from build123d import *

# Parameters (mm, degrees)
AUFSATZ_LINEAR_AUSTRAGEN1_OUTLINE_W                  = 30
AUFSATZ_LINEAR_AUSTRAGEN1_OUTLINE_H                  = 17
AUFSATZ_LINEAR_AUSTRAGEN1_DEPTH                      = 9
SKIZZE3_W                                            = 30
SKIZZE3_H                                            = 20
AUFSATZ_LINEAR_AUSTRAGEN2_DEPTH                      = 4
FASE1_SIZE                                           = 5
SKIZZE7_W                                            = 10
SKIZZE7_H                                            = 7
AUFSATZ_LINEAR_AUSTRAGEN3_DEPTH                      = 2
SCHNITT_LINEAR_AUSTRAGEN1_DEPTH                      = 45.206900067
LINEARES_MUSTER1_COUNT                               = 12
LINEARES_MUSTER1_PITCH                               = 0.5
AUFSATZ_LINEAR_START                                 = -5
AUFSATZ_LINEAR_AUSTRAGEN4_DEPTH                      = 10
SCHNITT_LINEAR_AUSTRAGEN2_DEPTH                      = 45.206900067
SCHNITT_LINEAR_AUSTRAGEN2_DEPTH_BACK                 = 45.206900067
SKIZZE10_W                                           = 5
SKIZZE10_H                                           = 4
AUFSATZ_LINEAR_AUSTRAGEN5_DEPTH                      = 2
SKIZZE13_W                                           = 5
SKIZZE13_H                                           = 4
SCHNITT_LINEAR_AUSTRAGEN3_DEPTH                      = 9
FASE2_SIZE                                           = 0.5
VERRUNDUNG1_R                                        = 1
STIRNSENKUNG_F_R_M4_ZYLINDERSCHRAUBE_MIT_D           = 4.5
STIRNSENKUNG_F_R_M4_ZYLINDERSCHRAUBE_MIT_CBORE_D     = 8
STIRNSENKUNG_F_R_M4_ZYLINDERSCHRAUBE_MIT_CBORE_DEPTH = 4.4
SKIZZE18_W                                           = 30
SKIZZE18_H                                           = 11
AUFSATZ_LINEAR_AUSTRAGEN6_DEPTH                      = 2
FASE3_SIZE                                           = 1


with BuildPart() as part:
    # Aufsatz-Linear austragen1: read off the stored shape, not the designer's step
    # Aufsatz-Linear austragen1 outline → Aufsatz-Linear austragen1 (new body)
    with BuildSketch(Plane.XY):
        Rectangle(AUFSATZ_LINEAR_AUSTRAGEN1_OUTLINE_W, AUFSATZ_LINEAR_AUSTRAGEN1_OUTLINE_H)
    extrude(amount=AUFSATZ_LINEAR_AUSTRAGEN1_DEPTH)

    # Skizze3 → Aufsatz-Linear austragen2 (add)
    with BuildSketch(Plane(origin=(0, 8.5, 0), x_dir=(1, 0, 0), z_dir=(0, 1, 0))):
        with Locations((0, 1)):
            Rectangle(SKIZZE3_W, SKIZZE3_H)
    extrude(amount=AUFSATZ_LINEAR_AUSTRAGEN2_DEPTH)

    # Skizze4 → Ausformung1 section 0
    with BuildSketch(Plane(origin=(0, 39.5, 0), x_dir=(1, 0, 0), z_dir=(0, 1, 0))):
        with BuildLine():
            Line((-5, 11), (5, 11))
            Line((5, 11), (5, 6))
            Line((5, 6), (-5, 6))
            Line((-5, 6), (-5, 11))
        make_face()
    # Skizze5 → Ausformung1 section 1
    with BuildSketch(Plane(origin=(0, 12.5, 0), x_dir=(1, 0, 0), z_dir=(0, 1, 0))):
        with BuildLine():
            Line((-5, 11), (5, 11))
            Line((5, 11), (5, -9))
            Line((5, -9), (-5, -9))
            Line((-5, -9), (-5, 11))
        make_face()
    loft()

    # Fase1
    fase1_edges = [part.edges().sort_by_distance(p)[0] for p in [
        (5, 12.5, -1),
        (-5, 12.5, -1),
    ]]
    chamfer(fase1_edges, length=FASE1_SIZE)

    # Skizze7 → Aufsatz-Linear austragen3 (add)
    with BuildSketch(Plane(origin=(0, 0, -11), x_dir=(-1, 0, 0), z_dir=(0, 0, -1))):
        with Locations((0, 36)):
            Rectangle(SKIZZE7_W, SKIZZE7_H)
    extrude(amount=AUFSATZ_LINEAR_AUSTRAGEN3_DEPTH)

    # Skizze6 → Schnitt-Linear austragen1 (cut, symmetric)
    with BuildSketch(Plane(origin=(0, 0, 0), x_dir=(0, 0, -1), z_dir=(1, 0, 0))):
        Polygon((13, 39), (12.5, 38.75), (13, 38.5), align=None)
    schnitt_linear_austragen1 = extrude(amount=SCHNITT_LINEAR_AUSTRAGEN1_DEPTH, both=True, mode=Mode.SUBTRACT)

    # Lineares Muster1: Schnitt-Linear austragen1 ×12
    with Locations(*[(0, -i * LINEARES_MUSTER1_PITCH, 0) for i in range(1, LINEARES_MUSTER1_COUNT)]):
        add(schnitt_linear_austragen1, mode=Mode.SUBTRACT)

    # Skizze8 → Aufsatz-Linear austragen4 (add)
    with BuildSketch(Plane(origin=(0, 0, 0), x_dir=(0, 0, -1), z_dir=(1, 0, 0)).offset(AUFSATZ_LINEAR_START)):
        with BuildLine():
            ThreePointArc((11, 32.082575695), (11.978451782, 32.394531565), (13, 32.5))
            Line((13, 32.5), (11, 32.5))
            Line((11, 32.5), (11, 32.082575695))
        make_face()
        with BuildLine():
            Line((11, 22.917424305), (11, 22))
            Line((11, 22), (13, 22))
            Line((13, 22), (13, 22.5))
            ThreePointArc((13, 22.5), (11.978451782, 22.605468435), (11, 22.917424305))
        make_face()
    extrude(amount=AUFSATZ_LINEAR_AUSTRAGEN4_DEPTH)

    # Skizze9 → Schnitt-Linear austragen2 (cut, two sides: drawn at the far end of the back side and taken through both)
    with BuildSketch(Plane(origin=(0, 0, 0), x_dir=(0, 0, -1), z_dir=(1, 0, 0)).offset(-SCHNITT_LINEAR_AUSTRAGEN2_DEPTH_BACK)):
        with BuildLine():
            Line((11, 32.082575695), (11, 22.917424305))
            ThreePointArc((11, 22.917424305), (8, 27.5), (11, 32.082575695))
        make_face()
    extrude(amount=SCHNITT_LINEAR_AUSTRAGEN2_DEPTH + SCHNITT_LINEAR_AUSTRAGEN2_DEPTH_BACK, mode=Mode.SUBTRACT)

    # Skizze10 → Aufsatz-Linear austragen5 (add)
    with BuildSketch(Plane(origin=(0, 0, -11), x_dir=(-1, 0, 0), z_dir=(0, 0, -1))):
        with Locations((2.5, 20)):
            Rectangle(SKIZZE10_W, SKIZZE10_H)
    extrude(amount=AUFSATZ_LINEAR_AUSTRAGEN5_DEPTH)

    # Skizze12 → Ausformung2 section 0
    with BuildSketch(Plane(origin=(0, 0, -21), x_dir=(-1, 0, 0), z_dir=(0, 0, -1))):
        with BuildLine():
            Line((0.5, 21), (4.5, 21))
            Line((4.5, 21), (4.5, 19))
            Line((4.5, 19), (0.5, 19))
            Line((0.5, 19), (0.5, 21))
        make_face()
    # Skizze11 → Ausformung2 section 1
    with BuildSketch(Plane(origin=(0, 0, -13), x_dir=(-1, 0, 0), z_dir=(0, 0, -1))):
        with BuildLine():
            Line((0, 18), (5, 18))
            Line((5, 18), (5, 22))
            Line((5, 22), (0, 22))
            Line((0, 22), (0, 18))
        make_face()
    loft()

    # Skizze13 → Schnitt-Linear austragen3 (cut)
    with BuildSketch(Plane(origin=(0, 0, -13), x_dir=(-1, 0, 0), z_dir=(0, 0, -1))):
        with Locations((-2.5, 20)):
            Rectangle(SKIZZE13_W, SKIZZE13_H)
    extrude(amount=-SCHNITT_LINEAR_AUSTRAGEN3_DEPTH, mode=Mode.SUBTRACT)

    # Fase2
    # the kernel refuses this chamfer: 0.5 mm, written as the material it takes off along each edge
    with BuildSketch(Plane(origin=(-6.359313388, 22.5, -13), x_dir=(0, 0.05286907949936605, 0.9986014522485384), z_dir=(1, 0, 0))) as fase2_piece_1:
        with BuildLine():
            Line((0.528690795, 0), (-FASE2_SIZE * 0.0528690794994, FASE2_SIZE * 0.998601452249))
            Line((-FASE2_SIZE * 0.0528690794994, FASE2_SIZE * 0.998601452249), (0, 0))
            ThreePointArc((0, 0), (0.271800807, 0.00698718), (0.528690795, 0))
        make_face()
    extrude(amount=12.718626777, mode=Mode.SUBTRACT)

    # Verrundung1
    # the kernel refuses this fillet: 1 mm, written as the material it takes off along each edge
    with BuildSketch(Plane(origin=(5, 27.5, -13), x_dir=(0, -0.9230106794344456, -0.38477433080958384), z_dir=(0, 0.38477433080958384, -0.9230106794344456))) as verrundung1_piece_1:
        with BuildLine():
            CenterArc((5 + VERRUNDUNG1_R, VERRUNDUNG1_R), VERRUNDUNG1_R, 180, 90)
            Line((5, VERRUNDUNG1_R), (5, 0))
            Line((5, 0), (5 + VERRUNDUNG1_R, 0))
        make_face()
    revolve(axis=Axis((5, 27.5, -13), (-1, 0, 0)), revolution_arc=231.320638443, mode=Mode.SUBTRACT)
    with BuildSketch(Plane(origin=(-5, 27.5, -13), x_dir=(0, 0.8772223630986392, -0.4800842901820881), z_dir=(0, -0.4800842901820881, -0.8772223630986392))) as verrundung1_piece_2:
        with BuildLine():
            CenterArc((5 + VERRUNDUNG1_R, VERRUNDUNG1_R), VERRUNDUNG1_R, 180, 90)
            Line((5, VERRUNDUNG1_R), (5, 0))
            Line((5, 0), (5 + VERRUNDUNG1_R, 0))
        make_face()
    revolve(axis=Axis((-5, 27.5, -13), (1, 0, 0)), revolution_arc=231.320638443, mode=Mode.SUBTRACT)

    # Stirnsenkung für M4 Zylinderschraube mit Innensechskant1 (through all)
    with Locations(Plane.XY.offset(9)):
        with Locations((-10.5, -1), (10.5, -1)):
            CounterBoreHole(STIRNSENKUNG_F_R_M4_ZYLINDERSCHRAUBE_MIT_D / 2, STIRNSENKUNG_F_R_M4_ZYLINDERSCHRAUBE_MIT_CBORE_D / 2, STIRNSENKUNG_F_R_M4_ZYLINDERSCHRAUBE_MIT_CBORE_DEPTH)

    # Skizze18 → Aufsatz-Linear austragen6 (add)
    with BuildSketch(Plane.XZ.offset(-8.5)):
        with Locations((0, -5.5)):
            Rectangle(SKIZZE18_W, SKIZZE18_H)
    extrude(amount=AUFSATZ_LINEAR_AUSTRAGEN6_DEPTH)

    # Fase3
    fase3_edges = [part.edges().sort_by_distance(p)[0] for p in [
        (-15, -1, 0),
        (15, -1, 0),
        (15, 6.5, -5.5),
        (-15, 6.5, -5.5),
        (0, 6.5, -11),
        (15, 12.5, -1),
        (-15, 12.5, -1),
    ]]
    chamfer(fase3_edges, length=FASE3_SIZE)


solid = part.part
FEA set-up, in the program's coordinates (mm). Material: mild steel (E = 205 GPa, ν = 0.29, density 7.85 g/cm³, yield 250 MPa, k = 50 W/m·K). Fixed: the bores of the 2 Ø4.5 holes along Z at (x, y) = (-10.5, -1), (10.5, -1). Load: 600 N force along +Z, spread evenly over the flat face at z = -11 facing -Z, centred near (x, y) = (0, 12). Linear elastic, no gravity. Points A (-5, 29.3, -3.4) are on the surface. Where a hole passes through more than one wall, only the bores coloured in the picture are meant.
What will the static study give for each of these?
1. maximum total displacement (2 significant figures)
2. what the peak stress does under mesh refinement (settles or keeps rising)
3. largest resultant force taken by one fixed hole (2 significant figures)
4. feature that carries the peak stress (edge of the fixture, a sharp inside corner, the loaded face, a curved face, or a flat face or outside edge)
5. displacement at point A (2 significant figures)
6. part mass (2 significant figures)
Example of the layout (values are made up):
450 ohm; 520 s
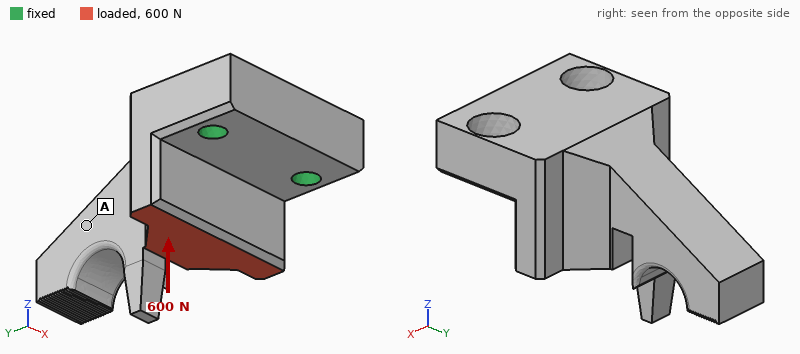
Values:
16 µm; keeps rising; 300 N; edge of the fixture; 11 µm; 85 g
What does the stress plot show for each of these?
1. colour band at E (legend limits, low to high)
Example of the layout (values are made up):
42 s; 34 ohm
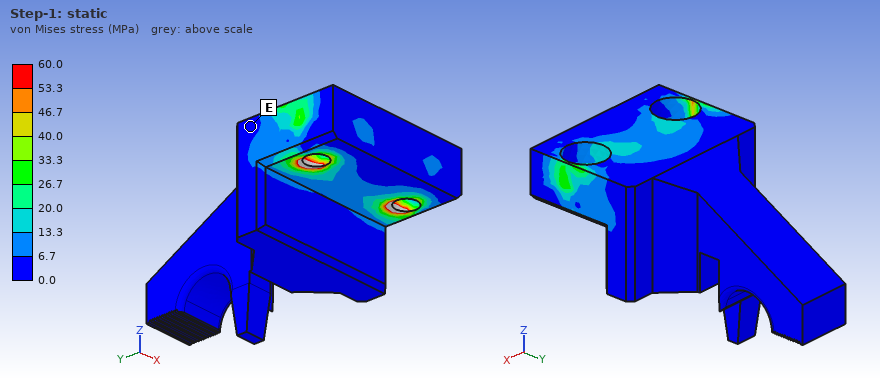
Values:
0.0 to 6.7 MPa
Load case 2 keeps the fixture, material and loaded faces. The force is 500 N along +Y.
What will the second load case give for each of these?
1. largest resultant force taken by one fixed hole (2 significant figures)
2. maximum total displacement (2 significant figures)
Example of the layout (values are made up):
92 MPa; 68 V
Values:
260 N; 20 µm
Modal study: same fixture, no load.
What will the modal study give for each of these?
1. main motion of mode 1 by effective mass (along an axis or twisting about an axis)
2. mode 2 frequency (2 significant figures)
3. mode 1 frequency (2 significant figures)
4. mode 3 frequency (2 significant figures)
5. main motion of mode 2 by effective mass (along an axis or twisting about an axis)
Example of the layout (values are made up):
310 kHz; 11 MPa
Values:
along Z; 9600 Hz; 4200 Hz; 17 kHz; along X
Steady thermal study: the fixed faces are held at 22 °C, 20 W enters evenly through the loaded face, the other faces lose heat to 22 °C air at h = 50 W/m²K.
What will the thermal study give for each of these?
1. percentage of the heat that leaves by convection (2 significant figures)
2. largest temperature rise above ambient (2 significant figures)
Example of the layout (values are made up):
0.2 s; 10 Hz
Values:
17 %; 37 K
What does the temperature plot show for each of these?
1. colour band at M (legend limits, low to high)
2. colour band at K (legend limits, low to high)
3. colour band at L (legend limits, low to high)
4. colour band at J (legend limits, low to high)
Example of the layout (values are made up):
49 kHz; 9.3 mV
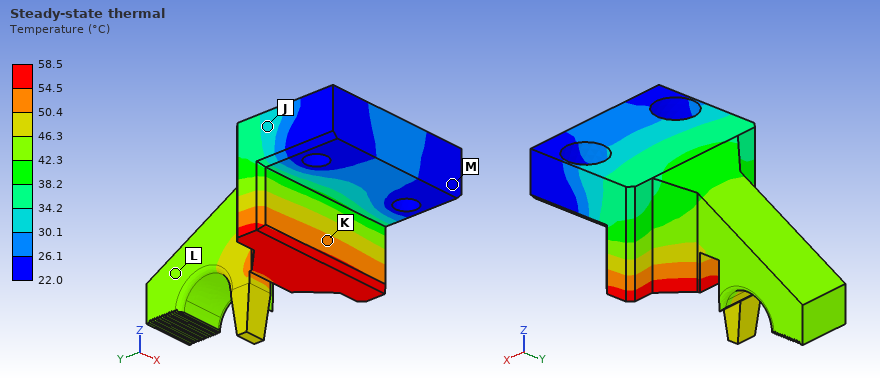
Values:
22.0 to 26.1 °C; 50.4 to 54.5 °C; 42.3 to 46.3 °C; 30.1 to 34.2 °C
